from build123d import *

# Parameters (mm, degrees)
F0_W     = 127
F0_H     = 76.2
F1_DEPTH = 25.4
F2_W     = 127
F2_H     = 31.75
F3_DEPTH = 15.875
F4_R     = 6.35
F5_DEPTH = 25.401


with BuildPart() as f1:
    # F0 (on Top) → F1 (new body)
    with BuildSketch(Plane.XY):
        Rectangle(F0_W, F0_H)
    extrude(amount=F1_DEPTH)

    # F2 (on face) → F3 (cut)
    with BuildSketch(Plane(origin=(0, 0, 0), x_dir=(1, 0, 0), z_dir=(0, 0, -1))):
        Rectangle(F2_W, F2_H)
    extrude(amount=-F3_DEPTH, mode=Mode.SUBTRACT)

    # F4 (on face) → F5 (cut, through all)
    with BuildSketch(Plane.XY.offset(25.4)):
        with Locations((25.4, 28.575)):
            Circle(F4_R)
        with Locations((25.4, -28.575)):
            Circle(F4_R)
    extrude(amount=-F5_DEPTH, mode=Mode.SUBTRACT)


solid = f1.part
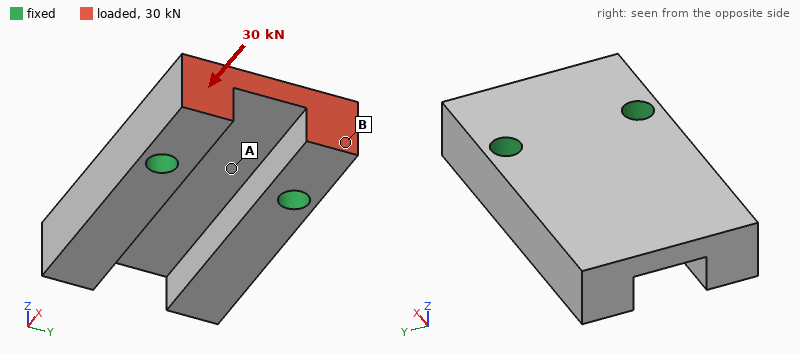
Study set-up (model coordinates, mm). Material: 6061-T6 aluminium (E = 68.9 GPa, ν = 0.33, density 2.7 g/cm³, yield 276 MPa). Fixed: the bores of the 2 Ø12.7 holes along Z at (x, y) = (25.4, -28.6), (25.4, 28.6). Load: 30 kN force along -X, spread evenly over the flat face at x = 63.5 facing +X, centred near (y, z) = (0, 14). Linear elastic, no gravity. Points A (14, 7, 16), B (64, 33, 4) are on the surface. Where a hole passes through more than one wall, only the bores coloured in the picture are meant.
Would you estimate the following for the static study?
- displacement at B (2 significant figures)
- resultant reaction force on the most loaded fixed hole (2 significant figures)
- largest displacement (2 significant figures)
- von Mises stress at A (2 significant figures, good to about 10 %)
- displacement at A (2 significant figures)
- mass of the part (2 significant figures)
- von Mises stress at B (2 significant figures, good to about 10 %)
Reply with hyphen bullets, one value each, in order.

- 10 µm
- 15 kN
- 15 µm
- 7.3 MPa
- 3.1 µm
- 470 g
- 21 MPa
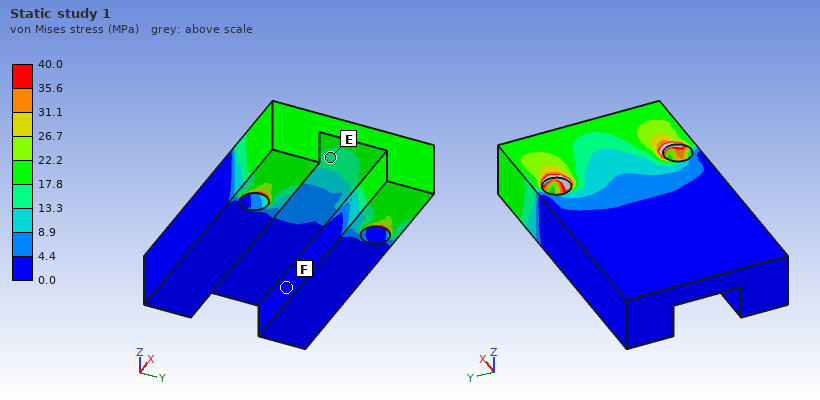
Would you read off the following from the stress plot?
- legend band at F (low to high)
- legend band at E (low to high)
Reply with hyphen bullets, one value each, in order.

- 0.0 to 4.4 MPa
- 13.3 to 17.8 MPa
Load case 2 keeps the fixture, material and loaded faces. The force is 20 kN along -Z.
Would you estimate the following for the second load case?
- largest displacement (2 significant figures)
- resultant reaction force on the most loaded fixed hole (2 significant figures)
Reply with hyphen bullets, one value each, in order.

- 0.12 mm
- 10 kN
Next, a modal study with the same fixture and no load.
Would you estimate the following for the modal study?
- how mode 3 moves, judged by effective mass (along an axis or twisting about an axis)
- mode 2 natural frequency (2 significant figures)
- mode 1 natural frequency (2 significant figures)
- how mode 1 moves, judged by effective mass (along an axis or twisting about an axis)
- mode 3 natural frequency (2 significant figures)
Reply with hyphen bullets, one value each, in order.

- along Y
- 3700 Hz
- 2600 Hz
- along Z
- 5800 Hz
